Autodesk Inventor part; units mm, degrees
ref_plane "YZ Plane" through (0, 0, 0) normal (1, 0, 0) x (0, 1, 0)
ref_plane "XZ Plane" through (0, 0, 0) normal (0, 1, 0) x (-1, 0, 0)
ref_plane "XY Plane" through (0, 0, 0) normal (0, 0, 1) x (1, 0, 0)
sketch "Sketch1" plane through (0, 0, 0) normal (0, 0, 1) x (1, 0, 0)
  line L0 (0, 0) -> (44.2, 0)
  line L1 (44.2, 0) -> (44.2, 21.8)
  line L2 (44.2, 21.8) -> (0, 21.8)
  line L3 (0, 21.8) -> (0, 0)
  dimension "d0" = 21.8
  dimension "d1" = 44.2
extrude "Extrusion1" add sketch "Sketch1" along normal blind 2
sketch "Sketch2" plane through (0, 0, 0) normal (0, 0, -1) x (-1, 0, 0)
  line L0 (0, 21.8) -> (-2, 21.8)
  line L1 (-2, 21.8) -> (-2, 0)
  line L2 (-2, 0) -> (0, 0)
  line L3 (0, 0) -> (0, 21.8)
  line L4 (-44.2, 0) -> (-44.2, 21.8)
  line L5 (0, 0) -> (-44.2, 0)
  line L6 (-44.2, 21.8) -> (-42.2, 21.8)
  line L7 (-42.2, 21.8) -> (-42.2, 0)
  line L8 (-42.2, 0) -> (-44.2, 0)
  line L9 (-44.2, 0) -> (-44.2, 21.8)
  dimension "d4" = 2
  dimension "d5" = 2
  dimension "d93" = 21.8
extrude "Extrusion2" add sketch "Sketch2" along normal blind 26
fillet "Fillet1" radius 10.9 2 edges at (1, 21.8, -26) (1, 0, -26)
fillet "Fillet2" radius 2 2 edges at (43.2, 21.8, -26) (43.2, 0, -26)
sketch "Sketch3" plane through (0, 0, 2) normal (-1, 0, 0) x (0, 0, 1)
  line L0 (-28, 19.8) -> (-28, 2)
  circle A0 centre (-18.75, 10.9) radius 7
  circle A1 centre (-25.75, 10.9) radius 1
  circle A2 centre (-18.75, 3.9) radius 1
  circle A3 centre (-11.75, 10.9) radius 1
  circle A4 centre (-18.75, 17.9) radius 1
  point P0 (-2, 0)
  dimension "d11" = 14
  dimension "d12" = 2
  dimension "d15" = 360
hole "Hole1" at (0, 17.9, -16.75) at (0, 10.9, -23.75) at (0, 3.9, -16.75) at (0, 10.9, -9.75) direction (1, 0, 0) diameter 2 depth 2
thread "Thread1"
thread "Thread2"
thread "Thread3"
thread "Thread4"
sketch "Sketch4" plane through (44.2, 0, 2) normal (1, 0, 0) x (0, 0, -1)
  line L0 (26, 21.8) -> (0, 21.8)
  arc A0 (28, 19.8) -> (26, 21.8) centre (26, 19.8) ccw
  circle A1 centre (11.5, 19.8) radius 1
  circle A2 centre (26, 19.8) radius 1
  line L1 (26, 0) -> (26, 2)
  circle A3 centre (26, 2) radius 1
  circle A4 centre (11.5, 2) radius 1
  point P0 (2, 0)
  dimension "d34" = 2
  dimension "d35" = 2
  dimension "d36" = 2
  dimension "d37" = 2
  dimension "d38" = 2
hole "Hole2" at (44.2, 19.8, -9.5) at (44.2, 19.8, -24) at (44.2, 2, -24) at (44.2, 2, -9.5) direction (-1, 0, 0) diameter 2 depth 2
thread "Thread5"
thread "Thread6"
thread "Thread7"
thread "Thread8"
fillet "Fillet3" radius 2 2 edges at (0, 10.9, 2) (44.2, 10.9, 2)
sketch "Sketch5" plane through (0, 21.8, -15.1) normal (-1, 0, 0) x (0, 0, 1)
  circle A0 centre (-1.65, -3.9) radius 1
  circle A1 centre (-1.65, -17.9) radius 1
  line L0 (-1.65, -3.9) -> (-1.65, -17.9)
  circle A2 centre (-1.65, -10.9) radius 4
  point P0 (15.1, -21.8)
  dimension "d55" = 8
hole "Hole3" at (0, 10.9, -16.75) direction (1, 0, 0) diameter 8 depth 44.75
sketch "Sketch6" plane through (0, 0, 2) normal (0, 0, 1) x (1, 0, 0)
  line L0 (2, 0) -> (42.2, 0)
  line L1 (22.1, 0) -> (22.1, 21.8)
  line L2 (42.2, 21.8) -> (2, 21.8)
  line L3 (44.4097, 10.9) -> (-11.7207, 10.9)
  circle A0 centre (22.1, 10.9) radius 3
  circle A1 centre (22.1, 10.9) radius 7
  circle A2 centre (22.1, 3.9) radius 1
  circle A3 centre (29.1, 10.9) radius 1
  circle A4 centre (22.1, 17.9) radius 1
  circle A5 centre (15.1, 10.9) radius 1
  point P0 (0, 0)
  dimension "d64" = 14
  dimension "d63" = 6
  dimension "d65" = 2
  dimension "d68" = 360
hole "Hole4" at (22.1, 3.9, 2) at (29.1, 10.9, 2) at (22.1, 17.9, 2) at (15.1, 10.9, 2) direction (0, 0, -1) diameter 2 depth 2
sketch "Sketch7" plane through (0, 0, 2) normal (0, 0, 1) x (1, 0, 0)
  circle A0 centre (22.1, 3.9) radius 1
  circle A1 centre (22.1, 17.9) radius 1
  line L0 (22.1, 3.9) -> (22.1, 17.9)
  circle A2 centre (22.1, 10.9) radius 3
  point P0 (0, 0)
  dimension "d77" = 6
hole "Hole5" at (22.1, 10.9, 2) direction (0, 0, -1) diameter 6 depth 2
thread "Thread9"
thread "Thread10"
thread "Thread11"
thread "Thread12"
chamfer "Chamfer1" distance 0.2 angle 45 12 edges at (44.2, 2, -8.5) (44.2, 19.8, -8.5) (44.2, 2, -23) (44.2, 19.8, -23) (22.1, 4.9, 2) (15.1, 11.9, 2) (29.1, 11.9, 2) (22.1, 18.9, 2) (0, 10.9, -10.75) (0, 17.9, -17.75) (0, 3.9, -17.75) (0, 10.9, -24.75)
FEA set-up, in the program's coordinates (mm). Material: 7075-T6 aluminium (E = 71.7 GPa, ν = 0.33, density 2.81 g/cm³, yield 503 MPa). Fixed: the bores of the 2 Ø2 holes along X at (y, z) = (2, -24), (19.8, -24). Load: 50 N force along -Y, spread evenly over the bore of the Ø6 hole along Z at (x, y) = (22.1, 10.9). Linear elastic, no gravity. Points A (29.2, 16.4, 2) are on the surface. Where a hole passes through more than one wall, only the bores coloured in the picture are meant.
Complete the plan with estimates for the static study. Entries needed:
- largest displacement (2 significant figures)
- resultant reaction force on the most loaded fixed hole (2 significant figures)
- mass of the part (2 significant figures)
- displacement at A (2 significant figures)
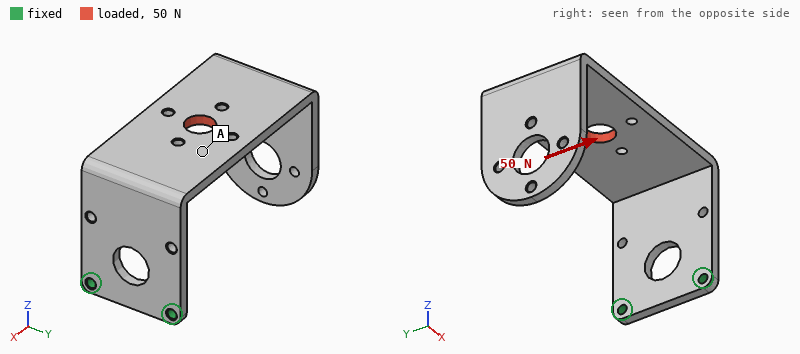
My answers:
0.66 mm
91 N
10 g
0.21 mm
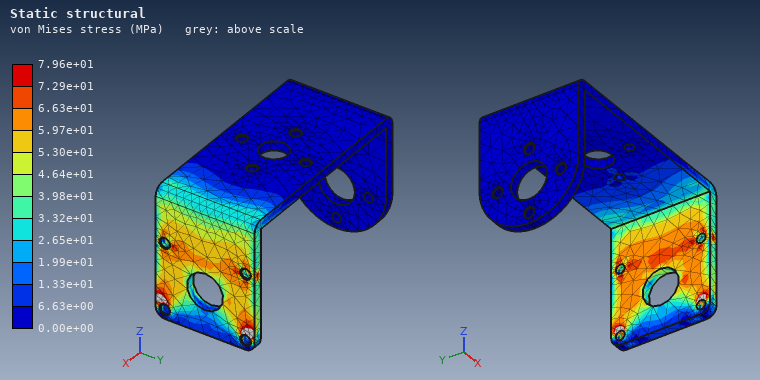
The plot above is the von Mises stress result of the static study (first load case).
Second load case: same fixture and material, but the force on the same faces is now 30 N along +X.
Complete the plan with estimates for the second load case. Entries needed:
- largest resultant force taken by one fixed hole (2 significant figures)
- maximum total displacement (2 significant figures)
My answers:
15 N
0.57 mm
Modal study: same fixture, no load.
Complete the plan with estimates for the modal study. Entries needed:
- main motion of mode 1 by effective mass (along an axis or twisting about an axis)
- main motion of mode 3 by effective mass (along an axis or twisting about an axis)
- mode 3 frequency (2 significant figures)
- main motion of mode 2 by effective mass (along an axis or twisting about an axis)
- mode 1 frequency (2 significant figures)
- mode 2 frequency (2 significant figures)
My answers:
along Z
along X
830 Hz
along Y
270 Hz
460 Hz
